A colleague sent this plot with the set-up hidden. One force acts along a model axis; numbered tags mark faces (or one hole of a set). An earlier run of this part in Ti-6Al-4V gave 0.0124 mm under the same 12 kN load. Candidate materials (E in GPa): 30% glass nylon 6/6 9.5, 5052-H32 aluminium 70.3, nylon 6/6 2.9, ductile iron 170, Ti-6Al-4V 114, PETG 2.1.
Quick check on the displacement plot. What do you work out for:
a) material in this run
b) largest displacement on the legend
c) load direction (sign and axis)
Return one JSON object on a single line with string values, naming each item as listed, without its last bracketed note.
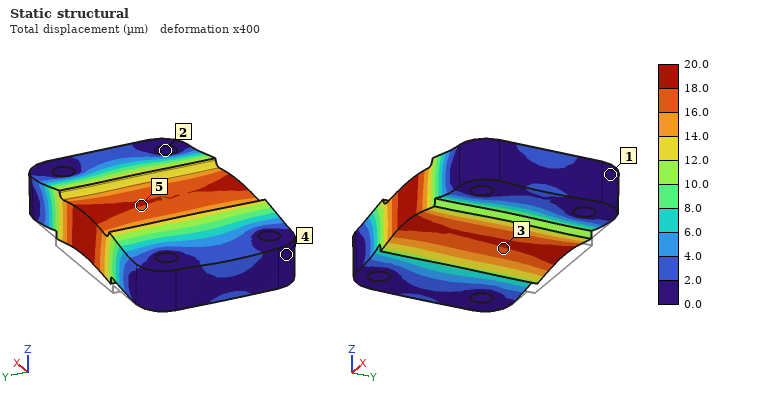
{"material in this run": "5052-H32 aluminium", "largest displacement on the legend": "20.0 µm", "load direction": "+Z"}
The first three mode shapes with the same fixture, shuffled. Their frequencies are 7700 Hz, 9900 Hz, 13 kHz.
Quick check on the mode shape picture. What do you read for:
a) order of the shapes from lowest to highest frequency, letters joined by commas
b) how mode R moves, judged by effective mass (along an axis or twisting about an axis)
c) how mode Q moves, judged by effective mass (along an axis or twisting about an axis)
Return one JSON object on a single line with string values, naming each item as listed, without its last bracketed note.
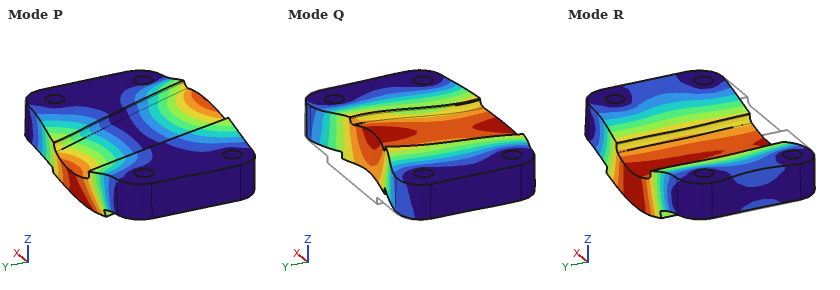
{"order of the shapes from lowest to highest frequency, letters joined by commas": "R, P, Q", "how mode R moves, judged by effective mass": "along Z", "how mode Q moves, judged by effective mass": "along Y"}
